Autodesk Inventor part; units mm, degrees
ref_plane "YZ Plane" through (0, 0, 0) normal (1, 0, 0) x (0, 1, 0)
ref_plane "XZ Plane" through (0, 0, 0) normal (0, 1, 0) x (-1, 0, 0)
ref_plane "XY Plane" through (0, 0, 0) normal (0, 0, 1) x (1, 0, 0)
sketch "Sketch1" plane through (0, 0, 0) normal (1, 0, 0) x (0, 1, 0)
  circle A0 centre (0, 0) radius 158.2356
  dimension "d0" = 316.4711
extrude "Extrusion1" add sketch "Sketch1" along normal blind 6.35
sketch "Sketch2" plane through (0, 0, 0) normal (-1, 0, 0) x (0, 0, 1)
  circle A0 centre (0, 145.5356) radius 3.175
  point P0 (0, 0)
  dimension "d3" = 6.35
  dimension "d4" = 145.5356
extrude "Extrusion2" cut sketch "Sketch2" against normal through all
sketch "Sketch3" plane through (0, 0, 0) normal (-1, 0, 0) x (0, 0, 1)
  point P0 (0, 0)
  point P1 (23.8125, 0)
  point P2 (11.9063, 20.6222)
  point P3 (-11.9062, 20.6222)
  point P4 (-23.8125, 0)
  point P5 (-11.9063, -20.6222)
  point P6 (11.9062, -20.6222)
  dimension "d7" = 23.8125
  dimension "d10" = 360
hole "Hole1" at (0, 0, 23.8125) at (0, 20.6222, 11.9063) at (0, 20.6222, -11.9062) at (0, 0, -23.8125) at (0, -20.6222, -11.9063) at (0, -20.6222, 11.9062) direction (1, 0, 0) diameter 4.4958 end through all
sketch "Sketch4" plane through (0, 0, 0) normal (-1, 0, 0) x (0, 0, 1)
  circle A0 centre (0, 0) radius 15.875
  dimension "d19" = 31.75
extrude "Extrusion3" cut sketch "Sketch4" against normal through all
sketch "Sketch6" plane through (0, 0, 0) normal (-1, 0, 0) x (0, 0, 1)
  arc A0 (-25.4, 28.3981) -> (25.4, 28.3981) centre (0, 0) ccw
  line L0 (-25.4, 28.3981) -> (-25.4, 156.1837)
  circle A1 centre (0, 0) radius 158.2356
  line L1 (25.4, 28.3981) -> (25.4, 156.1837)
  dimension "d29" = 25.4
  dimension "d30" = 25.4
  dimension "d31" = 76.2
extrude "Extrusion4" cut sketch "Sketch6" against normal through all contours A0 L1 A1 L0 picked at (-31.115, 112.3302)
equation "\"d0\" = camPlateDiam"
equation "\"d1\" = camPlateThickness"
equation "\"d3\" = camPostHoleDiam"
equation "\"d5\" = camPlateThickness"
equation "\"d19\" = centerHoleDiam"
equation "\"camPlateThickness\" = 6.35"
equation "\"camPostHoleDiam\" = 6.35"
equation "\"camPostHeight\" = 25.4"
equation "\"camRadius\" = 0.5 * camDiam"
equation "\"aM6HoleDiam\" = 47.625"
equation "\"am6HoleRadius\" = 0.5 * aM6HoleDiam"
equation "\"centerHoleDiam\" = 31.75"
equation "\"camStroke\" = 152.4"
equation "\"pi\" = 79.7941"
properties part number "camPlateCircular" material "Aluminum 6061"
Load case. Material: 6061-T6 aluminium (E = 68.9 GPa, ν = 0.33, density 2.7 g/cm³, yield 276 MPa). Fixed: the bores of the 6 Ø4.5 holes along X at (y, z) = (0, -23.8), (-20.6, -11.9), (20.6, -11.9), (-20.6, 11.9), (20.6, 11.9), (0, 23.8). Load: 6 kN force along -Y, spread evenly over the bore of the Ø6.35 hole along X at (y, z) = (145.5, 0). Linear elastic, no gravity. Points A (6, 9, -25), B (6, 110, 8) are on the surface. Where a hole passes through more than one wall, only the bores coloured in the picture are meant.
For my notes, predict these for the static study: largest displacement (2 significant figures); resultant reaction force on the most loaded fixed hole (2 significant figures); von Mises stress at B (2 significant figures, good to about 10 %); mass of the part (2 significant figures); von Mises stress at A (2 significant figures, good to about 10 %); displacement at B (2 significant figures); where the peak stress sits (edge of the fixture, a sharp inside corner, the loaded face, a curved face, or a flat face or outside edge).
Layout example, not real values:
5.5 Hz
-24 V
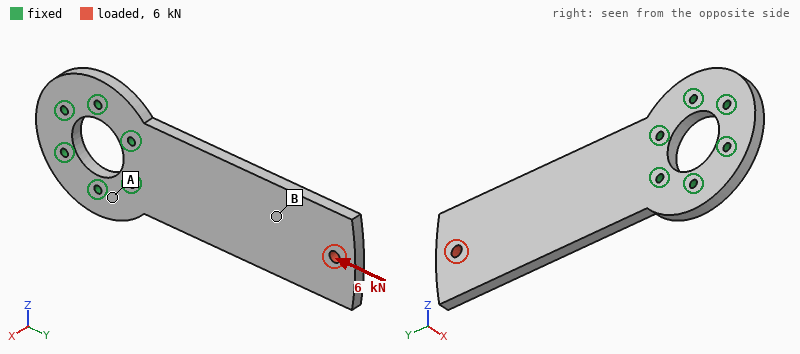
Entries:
45 µm
2.4 kN
20 MPa
170 g
7.1 MPa
25 µm
the loaded face
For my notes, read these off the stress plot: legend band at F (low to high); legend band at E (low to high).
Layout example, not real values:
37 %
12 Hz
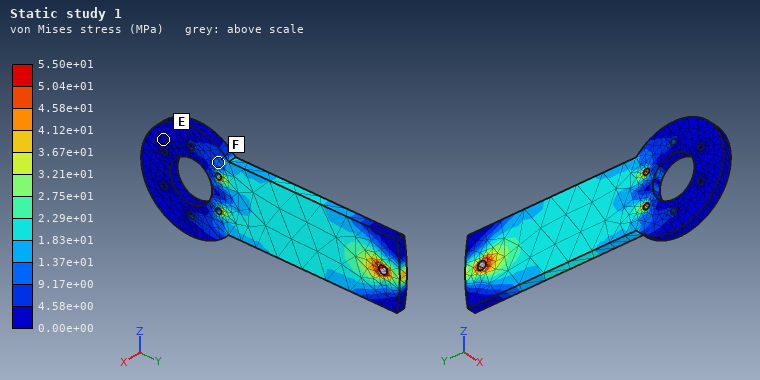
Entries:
9.17e+00 to 1.37e+01 MPa
0.00e+00 to 4.58e+00 MPa
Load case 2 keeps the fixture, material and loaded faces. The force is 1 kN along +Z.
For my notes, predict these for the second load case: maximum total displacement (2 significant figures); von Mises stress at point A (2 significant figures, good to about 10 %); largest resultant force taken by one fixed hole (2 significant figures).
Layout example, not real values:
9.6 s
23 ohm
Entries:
0.19 mm
15 MPa
2.4 kN
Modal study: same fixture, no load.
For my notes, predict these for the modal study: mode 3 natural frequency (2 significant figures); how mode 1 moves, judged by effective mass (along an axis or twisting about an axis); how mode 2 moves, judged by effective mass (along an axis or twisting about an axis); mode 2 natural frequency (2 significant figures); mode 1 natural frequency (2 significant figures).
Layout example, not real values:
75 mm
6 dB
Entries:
1700 Hz
along X
twisting about Y
1500 Hz
280 Hz
